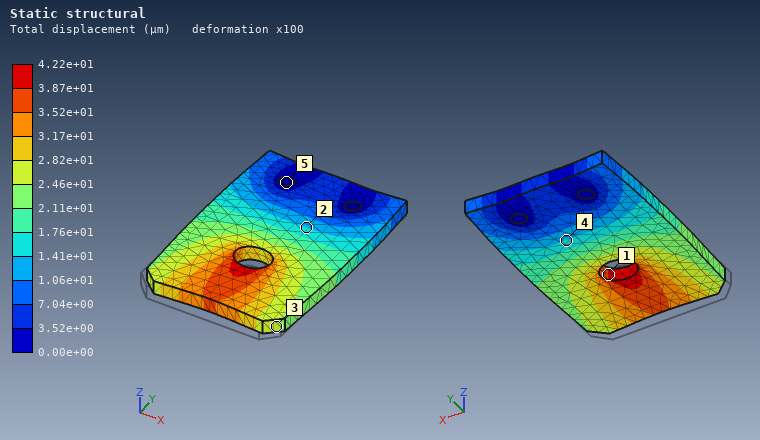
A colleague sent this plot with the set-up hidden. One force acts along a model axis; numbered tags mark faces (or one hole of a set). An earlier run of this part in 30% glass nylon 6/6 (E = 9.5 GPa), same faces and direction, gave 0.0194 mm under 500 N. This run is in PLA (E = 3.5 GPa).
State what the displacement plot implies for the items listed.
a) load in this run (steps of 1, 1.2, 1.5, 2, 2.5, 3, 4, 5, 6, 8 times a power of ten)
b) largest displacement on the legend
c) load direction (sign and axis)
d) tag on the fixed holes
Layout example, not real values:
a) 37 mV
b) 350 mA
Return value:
a) 400 N
b) 4.22e+01 µm
c) +Y
d) 5
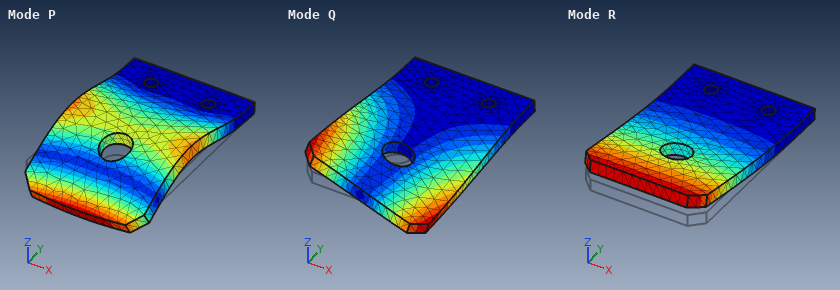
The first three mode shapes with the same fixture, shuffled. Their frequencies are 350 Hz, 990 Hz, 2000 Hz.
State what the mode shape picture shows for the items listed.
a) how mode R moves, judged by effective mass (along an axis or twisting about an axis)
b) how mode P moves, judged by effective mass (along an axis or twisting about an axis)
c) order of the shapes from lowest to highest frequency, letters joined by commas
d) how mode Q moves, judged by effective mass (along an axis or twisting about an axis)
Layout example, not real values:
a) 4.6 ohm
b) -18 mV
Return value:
a) along Z
b) along Z
c) R, Q, P
d) twisting about Y
